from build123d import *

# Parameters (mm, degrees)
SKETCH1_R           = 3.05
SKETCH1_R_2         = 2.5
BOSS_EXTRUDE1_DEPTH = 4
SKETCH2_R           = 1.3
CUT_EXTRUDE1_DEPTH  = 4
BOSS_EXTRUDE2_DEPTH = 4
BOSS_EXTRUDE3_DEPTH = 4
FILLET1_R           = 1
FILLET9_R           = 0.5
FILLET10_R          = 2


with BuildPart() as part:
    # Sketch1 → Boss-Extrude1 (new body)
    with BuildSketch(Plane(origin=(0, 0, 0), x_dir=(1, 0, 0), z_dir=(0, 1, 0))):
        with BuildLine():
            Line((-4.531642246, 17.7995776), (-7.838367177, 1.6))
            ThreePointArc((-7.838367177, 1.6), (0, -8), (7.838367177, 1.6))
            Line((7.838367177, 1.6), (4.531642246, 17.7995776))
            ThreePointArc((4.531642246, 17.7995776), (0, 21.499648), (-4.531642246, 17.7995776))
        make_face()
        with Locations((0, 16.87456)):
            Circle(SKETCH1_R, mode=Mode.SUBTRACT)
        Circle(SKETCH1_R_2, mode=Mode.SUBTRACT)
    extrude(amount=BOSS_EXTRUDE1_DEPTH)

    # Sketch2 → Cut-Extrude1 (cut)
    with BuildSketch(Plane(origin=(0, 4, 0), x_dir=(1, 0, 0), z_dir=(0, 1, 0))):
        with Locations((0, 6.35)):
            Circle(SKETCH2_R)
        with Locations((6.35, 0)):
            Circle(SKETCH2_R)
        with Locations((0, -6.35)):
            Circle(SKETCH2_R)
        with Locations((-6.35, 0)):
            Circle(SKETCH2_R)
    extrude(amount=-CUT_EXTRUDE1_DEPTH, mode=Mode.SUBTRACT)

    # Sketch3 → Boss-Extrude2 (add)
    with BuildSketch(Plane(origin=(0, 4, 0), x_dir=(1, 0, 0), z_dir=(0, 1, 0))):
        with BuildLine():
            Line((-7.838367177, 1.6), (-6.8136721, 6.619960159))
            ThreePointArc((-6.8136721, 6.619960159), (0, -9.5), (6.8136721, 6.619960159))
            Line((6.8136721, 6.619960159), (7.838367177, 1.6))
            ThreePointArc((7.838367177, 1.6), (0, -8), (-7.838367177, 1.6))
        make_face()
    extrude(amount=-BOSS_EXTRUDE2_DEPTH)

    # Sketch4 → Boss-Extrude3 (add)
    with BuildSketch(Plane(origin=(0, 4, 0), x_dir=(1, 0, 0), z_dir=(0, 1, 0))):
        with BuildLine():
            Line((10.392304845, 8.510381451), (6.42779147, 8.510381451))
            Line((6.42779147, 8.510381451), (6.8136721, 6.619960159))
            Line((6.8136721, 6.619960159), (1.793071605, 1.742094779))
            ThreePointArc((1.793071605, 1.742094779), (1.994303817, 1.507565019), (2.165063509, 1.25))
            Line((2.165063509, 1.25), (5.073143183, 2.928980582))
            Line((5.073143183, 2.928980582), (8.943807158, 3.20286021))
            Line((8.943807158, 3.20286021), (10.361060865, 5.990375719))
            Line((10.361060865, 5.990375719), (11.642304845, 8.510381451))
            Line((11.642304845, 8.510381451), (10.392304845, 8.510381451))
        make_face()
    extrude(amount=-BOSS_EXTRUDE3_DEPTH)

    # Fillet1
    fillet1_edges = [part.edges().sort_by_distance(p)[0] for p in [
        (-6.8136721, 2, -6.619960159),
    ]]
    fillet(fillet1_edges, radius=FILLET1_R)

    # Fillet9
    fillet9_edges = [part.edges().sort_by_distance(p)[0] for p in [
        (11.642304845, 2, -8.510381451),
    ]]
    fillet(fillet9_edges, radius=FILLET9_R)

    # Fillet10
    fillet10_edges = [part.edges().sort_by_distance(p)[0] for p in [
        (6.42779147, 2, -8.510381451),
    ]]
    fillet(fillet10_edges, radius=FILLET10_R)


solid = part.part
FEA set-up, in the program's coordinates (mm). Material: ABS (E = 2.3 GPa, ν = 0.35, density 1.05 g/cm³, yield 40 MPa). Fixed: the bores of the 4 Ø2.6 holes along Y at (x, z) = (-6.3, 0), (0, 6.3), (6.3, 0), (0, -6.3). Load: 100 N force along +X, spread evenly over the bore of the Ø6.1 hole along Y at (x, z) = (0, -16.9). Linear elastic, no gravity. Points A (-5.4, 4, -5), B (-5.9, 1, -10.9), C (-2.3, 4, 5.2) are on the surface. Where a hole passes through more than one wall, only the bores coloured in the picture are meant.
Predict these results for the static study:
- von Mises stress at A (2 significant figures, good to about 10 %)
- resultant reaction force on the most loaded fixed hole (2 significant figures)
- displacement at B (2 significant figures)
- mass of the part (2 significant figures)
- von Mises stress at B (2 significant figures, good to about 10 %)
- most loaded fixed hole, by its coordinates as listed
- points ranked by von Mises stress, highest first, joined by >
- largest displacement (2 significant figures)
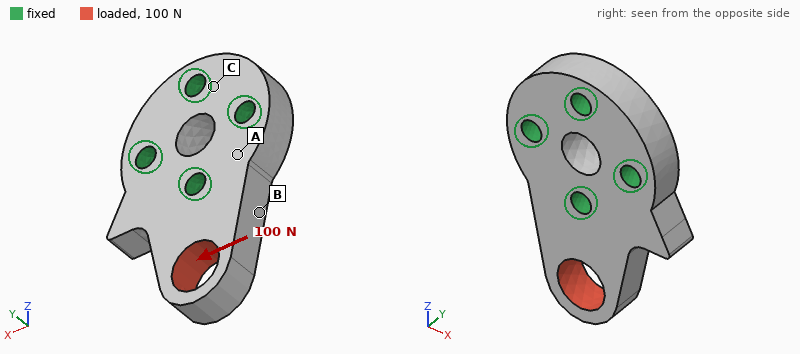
4.8 MPa
96 N
0.033 mm
1.5 g
8.9 MPa
(0, -6.3)
B > A > C
0.17 mm
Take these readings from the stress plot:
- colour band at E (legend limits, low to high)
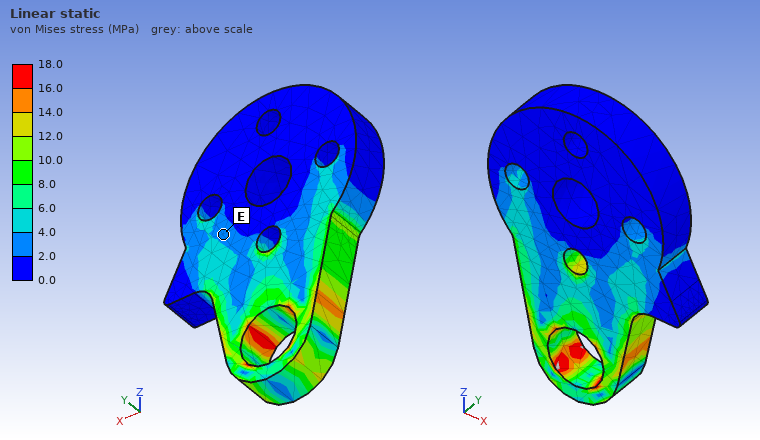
2.0 to 4.0 MPa
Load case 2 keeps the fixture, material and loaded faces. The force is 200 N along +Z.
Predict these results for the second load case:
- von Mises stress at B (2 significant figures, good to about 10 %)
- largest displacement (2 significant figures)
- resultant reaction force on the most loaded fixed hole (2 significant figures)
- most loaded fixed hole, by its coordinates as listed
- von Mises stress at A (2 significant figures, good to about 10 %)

5.4 MPa
70 µm
120 N
(0, -6.3)
2.6 MPa
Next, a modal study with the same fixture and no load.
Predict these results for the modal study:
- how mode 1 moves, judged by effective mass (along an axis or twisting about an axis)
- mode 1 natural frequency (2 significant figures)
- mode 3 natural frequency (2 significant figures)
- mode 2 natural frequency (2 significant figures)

along Y
6000 Hz
11 kHz
10 kHz
